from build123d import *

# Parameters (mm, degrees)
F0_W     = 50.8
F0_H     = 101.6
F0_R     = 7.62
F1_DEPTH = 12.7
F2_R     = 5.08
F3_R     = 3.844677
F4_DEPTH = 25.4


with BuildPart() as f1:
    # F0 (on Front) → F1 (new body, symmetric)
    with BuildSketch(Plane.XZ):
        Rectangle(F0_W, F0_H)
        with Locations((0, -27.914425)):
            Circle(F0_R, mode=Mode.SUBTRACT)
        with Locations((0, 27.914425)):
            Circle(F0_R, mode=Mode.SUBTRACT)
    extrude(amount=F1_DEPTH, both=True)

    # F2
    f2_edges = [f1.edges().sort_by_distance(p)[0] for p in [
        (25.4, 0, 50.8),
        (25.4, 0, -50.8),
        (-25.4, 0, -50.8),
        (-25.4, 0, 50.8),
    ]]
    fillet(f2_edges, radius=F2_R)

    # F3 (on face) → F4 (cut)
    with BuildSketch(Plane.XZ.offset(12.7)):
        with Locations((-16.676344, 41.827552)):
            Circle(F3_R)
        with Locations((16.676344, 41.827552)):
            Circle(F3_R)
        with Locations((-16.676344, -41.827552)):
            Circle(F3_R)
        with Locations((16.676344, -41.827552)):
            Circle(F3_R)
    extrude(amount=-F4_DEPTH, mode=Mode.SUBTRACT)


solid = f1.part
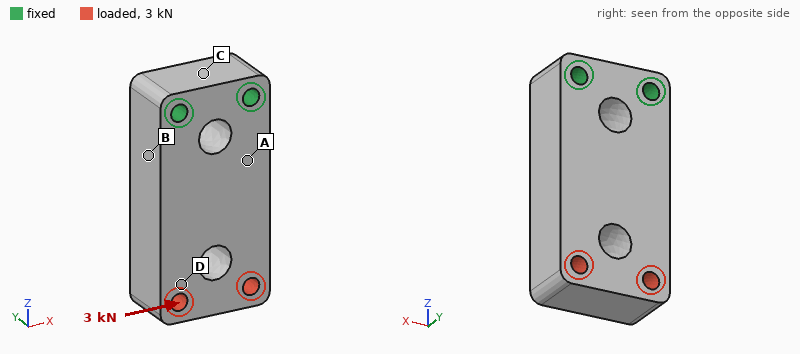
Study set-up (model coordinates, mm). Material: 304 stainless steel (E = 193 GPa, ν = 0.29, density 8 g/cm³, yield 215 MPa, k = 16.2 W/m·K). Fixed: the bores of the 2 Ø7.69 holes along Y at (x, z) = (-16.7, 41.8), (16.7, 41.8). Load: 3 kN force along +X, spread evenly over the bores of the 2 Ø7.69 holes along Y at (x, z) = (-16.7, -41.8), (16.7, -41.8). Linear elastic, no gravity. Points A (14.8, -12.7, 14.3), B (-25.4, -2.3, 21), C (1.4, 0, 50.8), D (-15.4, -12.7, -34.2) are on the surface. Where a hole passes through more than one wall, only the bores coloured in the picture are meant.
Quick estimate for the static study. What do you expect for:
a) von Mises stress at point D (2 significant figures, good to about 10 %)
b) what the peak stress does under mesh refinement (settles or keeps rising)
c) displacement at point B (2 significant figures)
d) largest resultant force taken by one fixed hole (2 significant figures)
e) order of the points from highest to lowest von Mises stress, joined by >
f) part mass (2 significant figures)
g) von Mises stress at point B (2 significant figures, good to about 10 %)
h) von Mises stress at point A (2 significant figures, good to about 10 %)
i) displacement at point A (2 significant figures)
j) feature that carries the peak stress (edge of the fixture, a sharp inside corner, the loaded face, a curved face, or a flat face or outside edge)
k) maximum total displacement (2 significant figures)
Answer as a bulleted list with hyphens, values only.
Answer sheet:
- 6.1 MPa
- keeps rising
- 3.5 µm
- 6.6 kN
- B > A > D > C
- 930 g
- 15 MPa
- 9.8 MPa
- 3.6 µm
- edge of the fixture
- 18 µm
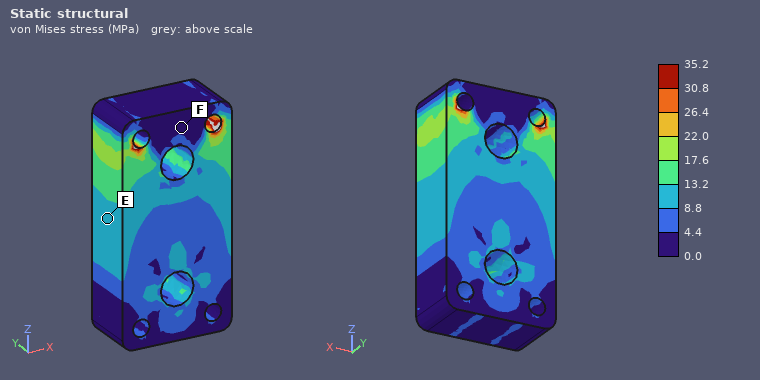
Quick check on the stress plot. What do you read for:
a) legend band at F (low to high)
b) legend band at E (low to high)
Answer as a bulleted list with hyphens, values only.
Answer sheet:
- 0.0 to 4.4 MPa
- 8.8 to 13.2 MPa
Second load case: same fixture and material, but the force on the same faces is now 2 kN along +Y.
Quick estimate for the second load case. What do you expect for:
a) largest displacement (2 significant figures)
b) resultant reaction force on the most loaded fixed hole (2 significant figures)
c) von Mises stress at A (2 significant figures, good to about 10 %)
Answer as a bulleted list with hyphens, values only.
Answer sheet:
- 44 µm
- 1.0 kN
- 24 MPa
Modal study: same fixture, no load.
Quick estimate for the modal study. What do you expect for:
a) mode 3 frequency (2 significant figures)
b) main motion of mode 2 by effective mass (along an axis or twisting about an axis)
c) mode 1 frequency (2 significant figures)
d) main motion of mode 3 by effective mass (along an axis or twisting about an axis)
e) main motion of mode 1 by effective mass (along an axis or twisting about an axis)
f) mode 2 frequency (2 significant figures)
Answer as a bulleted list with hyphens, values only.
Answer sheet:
- 6300 Hz
- along X
- 2200 Hz
- twisting about Z
- along Y
- 4000 Hz
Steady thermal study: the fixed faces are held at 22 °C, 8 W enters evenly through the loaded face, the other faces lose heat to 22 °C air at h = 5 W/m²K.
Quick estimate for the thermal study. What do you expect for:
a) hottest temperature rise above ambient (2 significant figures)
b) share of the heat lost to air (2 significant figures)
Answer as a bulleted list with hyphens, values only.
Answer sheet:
- 34 K
- 19 %
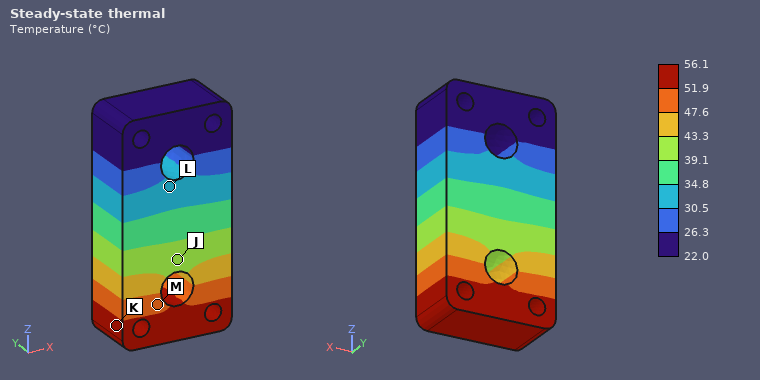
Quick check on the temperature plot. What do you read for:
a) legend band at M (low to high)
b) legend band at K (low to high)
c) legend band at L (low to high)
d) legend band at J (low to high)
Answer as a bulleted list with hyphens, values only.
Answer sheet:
- 47.6 to 51.9 °C
- 51.9 to 56.1 °C
- 30.5 to 34.8 °C
- 39.1 to 43.3 °C
